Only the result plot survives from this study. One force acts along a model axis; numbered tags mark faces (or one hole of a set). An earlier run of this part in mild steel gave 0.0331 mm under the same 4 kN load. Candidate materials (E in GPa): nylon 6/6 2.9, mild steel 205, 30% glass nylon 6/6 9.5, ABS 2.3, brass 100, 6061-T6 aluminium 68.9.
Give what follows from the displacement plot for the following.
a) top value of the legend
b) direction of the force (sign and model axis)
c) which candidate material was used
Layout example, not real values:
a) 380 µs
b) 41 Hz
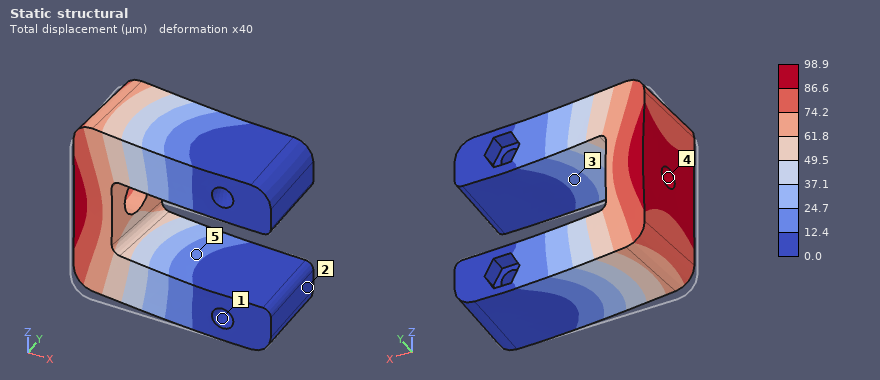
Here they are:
a) 98.9 µm
b) +Y
c) 6061-T6 aluminium
